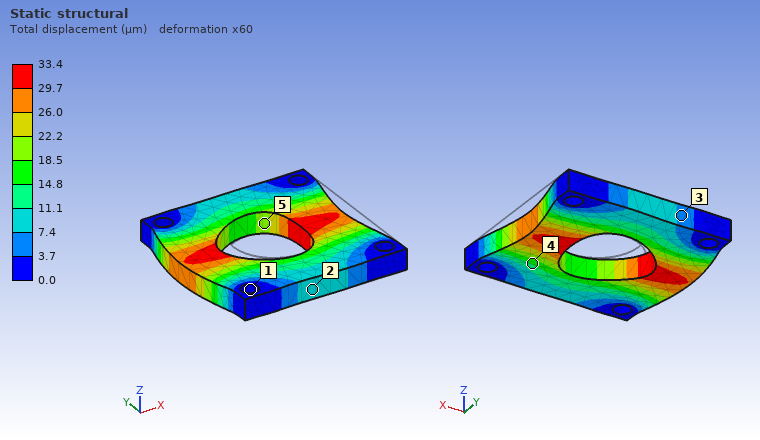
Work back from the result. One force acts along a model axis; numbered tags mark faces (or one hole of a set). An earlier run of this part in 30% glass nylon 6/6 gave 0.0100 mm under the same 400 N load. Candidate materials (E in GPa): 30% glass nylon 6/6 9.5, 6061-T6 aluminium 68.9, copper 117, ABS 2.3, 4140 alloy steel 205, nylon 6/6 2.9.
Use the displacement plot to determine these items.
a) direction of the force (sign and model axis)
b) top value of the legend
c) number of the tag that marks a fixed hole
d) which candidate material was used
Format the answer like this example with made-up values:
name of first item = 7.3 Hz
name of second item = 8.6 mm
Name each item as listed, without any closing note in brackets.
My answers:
direction of the force = -X
top value of the legend = 33.4 µm
number of the tag that marks a fixed hole = 1
which candidate material was used = nylon 6/6
